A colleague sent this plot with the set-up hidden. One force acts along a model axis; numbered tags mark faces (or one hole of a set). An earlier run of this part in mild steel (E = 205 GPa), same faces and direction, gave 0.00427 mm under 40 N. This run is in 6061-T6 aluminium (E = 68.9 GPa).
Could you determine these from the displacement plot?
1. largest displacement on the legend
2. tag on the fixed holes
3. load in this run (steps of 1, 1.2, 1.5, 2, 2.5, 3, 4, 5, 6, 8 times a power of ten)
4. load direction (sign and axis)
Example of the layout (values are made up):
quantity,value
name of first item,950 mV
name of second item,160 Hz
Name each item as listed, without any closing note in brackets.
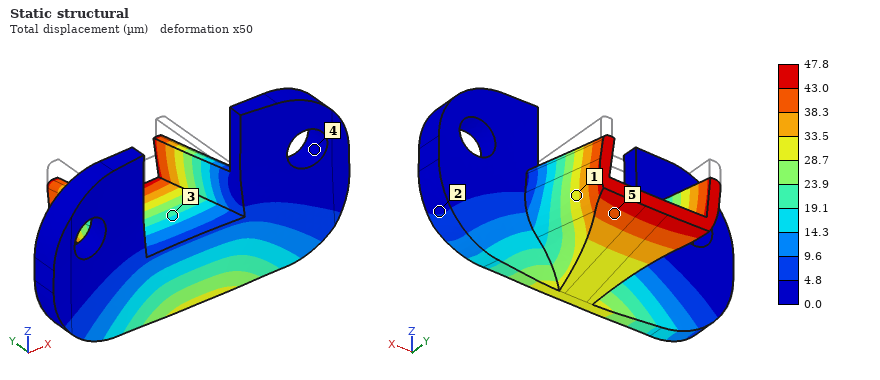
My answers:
quantity,value
largest displacement on the legend,47.8 µm
tag on the fixed holes,4
load in this run,150 N
load direction,-Z
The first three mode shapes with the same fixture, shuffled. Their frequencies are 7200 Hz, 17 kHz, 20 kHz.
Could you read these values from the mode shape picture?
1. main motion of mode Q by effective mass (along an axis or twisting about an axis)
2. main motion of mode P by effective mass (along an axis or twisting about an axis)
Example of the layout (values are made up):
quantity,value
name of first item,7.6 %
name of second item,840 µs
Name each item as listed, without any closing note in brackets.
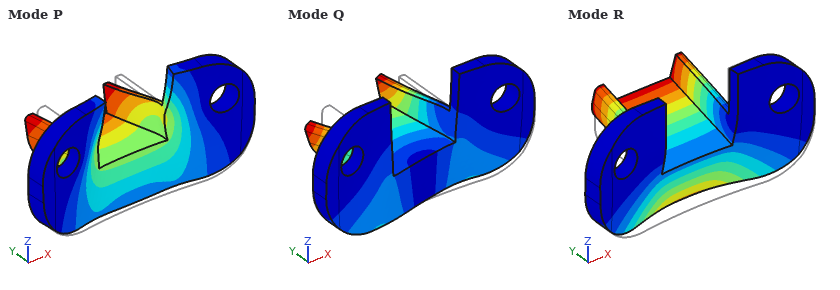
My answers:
quantity,value
main motion of mode Q by effective mass,along X
main motion of mode P by effective mass,along Y
